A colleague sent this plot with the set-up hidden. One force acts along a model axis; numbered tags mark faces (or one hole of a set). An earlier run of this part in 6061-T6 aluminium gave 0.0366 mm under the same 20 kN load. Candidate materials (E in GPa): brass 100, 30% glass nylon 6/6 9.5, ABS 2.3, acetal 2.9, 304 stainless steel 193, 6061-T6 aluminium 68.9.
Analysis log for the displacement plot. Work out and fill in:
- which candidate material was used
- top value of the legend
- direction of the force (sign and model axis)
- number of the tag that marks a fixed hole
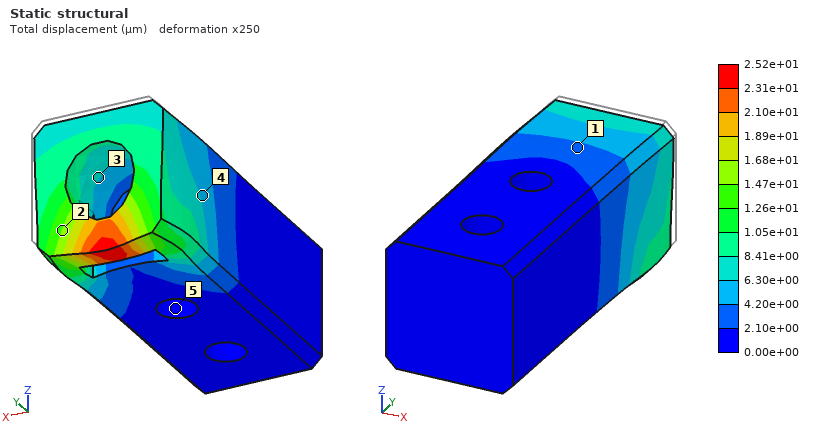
brass
2.52e+01 µm
-Y
5
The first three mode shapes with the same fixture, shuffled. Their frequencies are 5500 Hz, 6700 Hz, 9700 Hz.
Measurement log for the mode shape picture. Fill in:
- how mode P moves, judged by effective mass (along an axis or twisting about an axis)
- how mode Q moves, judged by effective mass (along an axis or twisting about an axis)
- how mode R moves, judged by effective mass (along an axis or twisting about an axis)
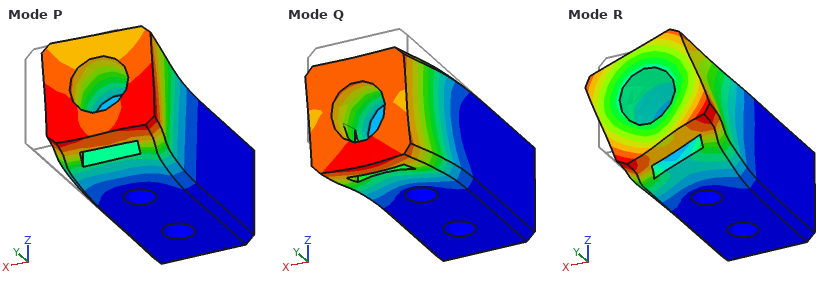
along X
along Z
twisting about Y
